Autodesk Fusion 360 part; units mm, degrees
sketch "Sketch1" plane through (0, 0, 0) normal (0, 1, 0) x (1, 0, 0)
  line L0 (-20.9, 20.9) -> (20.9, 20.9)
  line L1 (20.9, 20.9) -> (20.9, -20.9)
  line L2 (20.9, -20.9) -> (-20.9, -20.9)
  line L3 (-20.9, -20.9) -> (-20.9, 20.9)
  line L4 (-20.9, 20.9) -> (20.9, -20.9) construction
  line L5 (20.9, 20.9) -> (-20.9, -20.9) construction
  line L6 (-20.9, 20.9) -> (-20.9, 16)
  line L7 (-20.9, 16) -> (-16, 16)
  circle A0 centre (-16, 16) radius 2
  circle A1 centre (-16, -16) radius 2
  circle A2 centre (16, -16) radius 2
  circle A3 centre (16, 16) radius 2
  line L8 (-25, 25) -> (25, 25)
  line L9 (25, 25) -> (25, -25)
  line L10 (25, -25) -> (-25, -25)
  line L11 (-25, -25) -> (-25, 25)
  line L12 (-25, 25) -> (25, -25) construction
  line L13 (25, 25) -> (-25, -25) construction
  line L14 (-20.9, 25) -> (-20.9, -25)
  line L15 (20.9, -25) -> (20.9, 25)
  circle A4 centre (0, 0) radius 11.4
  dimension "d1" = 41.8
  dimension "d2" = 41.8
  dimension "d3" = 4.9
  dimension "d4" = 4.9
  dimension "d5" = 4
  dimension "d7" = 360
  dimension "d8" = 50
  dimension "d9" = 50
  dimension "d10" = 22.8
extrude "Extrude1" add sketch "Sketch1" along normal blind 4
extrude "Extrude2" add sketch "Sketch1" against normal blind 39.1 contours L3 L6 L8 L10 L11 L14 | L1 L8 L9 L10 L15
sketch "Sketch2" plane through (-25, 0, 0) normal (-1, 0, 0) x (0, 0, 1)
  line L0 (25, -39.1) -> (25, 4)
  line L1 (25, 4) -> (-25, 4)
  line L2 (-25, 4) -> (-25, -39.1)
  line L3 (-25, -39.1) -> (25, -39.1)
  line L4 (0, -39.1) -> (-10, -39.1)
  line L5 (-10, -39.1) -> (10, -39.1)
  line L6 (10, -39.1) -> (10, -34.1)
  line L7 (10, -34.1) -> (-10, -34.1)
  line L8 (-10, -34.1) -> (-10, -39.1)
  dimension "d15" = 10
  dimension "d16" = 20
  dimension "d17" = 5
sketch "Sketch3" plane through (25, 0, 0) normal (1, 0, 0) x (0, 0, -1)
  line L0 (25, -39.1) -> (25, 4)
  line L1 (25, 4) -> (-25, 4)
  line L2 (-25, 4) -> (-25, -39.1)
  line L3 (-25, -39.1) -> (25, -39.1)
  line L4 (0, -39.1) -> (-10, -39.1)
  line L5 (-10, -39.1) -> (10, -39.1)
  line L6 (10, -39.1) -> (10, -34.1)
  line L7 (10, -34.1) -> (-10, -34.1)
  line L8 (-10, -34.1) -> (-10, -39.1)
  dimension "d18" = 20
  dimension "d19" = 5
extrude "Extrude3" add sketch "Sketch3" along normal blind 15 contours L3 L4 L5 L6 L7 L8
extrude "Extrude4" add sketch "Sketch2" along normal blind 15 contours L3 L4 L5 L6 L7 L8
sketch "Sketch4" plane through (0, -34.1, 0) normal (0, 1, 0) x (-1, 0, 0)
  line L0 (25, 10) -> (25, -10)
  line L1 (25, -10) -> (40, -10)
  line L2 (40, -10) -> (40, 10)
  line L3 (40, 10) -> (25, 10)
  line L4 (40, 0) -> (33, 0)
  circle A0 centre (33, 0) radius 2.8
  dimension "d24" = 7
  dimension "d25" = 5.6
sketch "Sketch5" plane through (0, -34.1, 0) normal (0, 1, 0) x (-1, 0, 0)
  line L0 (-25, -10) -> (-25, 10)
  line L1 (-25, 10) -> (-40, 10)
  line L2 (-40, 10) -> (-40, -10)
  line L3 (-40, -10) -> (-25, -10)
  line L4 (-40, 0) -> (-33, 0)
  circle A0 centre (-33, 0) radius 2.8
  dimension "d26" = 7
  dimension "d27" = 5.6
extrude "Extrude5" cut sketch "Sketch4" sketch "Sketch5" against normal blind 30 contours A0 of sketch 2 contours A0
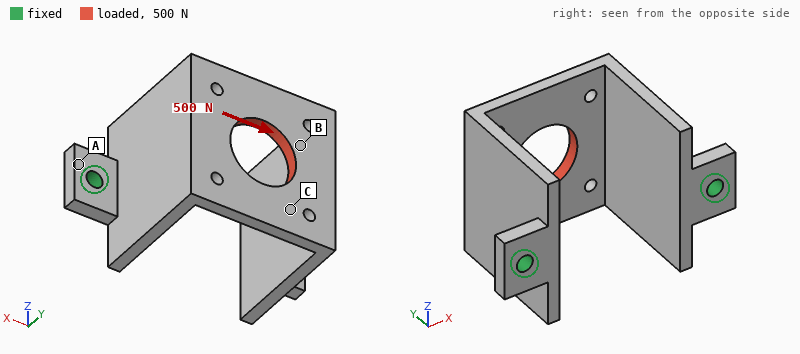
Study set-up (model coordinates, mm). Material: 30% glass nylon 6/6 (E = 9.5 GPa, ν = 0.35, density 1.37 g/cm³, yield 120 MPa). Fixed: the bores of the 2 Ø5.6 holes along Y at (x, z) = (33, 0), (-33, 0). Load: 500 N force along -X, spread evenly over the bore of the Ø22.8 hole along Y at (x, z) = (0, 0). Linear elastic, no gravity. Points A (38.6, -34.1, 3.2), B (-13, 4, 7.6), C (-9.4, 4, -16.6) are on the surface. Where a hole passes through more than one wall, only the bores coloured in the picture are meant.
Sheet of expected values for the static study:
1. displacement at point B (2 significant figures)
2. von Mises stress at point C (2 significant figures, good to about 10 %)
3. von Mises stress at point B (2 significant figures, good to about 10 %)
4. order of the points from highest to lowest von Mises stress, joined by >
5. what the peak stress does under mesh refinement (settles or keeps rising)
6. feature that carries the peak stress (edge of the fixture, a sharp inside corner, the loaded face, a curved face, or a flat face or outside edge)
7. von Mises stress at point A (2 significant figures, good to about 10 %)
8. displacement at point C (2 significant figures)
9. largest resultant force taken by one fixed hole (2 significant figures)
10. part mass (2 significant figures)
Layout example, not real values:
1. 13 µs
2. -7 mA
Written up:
1. 1.0 mm
2. 19 MPa
3. 27 MPa
4. B > C > A
5. keeps rising
6. edge of the fixture
7. 6.9 MPa
8. 1.00 mm
9. 330 N
10. 37 g
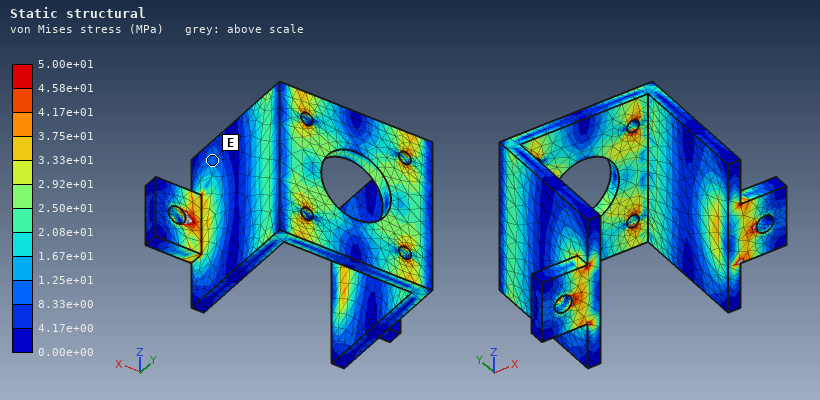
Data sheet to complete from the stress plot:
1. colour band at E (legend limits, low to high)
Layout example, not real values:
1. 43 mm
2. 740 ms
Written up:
1. 8.33e+00 to 1.25e+01 MPa
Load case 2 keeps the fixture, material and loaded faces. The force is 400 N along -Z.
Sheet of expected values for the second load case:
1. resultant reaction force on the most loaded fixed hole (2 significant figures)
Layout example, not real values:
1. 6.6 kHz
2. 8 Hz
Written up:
1. 200 N
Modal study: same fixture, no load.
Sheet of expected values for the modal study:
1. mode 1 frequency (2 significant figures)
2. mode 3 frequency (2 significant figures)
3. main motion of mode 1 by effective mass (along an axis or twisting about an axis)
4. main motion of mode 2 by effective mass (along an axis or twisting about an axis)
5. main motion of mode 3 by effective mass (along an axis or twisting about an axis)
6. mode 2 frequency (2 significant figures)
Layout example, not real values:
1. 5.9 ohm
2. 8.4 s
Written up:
1. 750 Hz
2. 1100 Hz
3. along Z
4. along X
5. twisting about Y
6. 830 Hz
